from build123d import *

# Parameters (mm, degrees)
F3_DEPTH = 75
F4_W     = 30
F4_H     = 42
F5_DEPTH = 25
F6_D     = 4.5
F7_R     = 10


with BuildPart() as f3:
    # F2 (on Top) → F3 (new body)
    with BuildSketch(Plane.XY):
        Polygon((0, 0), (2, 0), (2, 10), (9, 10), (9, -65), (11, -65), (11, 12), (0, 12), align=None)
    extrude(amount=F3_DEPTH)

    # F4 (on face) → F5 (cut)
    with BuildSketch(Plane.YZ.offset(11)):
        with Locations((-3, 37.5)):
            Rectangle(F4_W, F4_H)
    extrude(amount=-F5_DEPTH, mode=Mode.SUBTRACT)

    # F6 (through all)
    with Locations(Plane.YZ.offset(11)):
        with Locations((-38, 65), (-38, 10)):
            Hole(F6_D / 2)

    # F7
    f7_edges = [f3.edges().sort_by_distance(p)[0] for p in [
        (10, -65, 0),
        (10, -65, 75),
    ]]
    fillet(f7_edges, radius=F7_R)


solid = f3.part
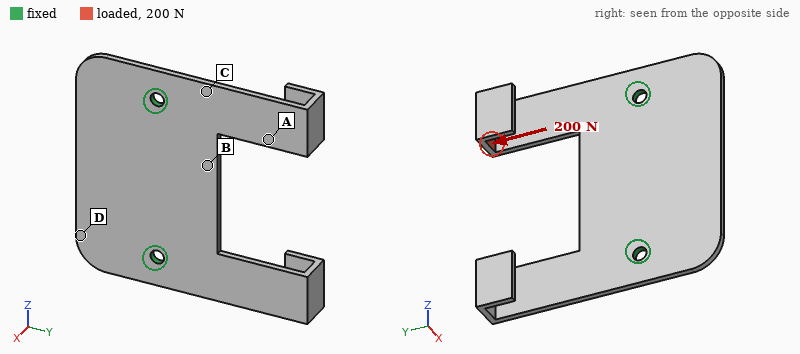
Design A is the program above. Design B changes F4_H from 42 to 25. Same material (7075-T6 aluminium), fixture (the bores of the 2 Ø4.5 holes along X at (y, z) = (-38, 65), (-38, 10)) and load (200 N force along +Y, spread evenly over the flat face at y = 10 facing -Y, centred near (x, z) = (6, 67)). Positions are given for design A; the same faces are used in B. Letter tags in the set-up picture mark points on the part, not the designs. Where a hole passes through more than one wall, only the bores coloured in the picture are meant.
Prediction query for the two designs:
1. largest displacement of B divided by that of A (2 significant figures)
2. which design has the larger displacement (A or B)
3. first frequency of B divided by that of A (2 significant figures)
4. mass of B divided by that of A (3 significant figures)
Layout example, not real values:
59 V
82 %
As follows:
0.72
A
0.90
1.16
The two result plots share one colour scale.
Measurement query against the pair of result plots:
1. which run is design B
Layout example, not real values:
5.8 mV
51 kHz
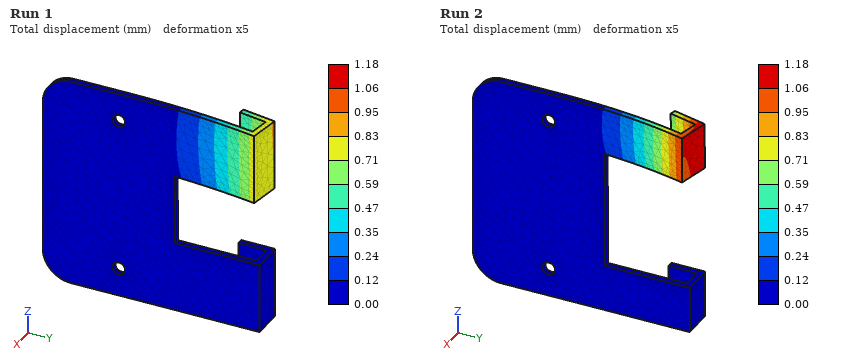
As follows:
Run 1
